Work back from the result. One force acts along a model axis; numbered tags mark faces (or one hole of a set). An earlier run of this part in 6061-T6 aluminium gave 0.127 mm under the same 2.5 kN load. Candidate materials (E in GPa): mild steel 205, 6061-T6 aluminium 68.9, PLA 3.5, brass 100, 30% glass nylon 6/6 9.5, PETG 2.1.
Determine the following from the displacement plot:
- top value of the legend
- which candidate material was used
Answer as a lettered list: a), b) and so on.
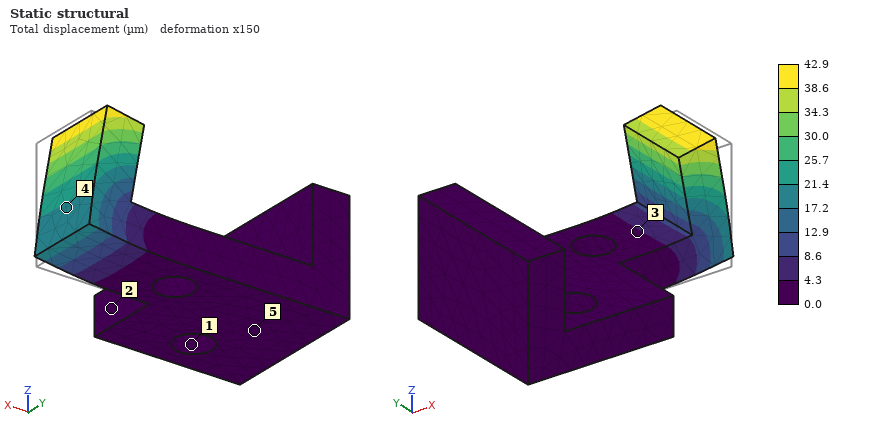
a) 42.9 µm
b) mild steel
